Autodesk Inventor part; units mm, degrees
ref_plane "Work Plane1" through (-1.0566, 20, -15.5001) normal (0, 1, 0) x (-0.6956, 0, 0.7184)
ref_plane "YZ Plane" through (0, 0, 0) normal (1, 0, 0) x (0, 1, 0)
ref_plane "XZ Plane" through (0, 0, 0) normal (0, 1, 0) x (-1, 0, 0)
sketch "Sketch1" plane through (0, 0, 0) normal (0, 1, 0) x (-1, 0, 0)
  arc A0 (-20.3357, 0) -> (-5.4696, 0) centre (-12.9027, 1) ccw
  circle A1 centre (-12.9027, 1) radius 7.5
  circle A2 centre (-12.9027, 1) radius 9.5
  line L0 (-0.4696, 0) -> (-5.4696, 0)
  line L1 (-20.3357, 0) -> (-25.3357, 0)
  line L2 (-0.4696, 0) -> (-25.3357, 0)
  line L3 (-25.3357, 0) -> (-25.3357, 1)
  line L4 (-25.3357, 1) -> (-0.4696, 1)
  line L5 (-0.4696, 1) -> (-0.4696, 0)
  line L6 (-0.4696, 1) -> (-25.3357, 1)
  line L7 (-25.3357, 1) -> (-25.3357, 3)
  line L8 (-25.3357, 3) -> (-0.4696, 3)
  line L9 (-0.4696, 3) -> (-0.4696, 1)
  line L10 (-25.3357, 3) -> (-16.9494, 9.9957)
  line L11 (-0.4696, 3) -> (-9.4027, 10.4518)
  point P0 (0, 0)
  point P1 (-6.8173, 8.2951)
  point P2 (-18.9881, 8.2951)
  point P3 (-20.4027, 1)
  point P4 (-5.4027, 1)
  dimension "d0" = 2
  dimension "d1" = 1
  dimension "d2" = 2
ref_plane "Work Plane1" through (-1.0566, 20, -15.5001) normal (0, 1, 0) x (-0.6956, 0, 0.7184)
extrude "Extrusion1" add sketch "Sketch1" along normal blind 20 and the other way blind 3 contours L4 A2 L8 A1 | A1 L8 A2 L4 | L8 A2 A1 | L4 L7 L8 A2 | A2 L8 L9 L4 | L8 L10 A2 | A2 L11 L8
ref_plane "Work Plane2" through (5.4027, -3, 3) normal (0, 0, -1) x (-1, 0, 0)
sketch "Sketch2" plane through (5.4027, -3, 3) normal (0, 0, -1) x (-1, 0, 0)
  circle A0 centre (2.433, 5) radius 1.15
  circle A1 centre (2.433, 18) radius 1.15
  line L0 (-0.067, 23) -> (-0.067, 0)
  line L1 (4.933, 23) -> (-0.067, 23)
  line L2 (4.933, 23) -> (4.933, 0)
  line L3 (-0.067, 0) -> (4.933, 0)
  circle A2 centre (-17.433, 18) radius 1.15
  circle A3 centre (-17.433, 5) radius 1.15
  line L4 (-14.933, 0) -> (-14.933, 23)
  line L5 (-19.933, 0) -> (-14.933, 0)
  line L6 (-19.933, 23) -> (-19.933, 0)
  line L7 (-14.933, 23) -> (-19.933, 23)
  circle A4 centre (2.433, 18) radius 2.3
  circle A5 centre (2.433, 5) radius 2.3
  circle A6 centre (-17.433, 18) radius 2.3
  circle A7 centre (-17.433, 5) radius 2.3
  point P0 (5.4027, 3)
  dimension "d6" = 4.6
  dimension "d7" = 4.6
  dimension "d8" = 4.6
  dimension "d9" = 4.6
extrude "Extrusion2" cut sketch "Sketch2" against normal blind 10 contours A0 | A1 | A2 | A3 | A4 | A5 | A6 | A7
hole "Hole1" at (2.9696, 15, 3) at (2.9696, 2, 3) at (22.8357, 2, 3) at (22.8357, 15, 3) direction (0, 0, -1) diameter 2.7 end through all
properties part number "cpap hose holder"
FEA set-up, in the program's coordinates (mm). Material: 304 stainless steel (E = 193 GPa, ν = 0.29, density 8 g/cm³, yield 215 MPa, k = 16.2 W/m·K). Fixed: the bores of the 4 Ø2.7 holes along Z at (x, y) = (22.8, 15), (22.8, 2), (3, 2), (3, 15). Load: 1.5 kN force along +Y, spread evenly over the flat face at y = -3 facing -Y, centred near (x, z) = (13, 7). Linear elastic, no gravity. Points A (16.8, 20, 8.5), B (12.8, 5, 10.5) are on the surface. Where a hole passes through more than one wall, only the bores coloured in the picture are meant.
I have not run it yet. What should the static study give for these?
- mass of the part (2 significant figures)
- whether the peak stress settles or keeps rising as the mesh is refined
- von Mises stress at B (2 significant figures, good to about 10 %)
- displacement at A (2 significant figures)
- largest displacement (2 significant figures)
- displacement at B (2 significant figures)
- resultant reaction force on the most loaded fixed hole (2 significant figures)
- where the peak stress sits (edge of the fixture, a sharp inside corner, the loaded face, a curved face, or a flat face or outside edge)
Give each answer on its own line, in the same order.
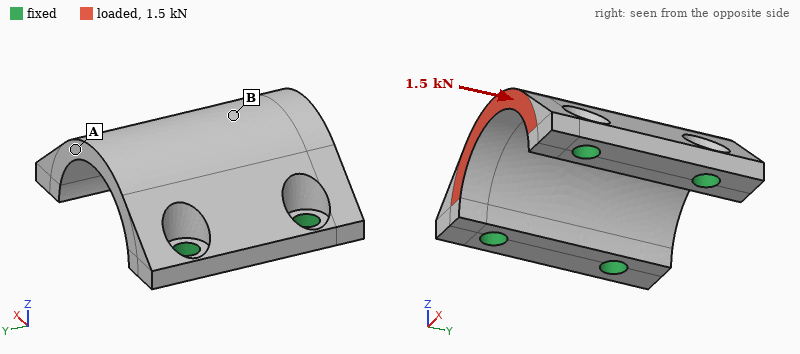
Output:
13 g
keeps rising
28 MPa
3.0 µm
6.4 µm
4.0 µm
530 N
edge of the fixture
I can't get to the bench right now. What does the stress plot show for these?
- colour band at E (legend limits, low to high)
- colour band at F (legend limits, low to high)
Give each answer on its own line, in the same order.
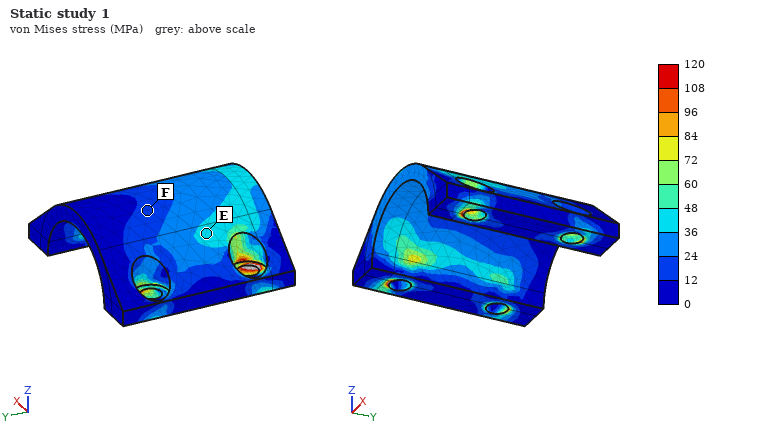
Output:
36 to 48 MPa
12 to 24 MPa
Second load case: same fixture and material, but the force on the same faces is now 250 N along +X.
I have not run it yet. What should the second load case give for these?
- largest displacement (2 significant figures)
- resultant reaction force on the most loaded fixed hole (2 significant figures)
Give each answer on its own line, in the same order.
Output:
3.2 µm
99 N
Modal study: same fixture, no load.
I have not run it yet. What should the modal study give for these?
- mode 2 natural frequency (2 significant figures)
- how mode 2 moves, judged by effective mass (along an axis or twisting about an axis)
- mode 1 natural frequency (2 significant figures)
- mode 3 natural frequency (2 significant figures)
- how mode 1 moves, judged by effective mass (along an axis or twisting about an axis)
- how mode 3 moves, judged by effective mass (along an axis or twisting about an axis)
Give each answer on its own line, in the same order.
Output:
35 kHz
along Y
29 kHz
39 kHz
along X
twisting about Z
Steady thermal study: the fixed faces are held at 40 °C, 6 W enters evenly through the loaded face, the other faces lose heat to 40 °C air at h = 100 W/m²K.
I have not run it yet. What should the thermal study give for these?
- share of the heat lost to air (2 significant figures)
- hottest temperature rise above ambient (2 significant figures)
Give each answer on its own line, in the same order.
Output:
34 %
65 K
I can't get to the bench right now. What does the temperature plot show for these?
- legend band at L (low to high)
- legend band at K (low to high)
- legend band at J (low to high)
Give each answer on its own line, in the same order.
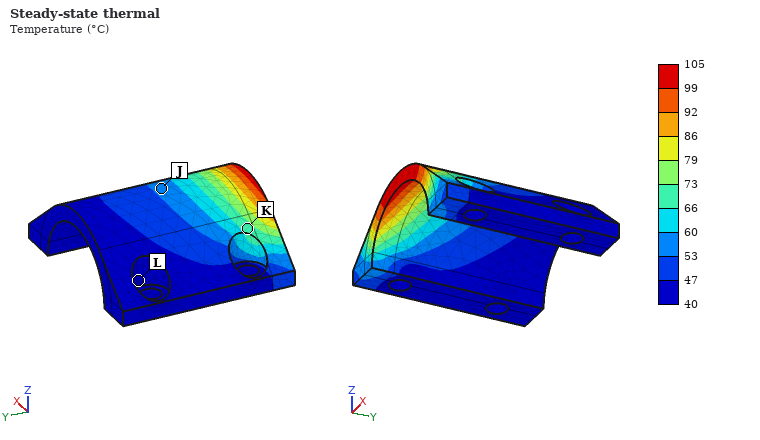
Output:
40 to 47 °C
66 to 73 °C
53 to 60 °C
